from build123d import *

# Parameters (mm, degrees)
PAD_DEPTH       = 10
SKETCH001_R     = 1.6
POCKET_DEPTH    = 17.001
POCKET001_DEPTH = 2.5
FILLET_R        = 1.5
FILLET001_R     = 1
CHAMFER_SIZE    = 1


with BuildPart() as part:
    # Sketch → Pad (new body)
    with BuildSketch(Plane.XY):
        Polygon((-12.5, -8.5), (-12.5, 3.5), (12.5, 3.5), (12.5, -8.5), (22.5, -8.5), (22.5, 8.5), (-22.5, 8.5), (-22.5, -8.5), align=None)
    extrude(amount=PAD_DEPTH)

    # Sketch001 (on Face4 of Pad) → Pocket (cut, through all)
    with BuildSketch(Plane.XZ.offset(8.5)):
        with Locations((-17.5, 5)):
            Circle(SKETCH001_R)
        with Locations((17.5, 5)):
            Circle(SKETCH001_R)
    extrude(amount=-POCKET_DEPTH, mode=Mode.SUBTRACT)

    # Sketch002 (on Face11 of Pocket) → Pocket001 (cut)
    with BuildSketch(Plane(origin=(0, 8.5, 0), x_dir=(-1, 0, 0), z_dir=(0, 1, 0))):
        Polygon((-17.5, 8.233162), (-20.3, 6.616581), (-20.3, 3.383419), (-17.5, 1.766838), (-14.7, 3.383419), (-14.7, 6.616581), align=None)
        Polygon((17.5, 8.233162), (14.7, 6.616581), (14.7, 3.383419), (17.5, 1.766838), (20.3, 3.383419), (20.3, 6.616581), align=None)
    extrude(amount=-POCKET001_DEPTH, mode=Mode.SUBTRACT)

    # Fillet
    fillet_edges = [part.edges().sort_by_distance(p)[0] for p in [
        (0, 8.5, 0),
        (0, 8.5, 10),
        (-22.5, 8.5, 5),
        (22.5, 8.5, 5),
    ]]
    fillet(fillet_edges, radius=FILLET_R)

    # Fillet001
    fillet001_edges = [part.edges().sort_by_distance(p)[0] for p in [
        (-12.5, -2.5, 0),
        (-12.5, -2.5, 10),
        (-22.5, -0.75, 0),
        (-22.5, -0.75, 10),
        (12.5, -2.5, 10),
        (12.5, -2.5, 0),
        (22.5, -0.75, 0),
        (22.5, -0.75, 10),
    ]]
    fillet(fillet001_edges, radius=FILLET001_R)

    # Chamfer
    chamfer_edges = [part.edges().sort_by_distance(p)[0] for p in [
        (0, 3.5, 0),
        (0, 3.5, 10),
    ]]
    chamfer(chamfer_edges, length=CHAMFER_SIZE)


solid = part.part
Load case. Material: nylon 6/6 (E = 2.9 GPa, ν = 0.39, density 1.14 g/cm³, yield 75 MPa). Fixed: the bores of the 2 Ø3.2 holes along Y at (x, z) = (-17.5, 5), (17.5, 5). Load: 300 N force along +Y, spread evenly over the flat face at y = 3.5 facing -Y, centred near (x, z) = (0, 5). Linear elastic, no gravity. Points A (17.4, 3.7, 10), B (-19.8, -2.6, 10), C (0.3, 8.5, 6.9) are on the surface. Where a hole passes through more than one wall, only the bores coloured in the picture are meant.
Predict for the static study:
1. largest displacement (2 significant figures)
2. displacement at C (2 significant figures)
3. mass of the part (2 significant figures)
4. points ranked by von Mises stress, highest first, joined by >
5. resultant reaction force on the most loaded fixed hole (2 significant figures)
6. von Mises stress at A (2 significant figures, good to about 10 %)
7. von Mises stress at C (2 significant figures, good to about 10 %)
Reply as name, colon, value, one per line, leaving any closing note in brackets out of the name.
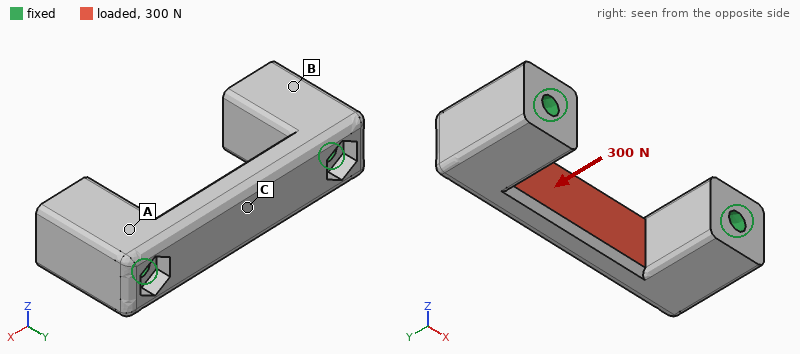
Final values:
largest displacement: 0.13 mm
displacement at C: 0.12 mm
mass of the part: 4.8 g
points ranked by von Mises stress, highest first, joined by >: C > A > B
resultant reaction force on the most loaded fixed hole: 170 N
von Mises stress at A: 3.1 MPa
von Mises stress at C: 14 MPa
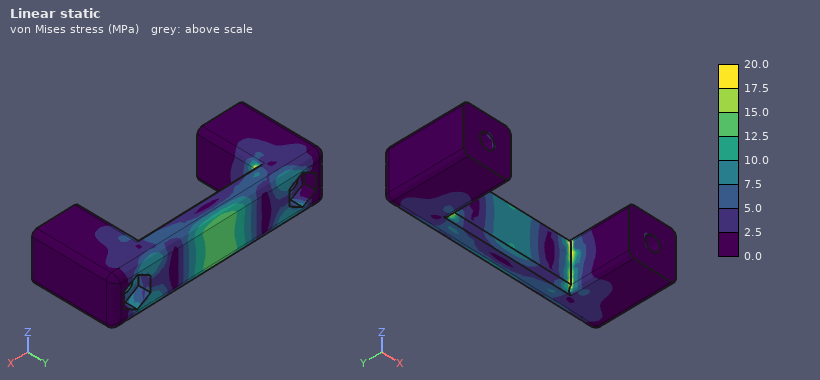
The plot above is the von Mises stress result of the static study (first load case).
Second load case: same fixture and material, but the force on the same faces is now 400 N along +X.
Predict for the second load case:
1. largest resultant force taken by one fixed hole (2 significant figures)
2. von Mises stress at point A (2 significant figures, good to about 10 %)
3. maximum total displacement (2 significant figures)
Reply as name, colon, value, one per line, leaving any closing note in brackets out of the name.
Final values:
largest resultant force taken by one fixed hole: 200 N
von Mises stress at point A: 1.8 MPa
maximum total displacement: 29 µm
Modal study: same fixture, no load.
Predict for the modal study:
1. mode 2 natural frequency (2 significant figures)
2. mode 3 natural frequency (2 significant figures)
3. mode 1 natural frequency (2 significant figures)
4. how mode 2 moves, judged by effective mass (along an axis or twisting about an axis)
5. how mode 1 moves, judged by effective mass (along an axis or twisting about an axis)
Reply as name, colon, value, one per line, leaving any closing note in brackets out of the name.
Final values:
mode 2 natural frequency: 8300 Hz
mode 3 natural frequency: 13 kHz
mode 1 natural frequency: 7400 Hz
how mode 2 moves, judged by effective mass: along Z
how mode 1 moves, judged by effective mass: along Y
